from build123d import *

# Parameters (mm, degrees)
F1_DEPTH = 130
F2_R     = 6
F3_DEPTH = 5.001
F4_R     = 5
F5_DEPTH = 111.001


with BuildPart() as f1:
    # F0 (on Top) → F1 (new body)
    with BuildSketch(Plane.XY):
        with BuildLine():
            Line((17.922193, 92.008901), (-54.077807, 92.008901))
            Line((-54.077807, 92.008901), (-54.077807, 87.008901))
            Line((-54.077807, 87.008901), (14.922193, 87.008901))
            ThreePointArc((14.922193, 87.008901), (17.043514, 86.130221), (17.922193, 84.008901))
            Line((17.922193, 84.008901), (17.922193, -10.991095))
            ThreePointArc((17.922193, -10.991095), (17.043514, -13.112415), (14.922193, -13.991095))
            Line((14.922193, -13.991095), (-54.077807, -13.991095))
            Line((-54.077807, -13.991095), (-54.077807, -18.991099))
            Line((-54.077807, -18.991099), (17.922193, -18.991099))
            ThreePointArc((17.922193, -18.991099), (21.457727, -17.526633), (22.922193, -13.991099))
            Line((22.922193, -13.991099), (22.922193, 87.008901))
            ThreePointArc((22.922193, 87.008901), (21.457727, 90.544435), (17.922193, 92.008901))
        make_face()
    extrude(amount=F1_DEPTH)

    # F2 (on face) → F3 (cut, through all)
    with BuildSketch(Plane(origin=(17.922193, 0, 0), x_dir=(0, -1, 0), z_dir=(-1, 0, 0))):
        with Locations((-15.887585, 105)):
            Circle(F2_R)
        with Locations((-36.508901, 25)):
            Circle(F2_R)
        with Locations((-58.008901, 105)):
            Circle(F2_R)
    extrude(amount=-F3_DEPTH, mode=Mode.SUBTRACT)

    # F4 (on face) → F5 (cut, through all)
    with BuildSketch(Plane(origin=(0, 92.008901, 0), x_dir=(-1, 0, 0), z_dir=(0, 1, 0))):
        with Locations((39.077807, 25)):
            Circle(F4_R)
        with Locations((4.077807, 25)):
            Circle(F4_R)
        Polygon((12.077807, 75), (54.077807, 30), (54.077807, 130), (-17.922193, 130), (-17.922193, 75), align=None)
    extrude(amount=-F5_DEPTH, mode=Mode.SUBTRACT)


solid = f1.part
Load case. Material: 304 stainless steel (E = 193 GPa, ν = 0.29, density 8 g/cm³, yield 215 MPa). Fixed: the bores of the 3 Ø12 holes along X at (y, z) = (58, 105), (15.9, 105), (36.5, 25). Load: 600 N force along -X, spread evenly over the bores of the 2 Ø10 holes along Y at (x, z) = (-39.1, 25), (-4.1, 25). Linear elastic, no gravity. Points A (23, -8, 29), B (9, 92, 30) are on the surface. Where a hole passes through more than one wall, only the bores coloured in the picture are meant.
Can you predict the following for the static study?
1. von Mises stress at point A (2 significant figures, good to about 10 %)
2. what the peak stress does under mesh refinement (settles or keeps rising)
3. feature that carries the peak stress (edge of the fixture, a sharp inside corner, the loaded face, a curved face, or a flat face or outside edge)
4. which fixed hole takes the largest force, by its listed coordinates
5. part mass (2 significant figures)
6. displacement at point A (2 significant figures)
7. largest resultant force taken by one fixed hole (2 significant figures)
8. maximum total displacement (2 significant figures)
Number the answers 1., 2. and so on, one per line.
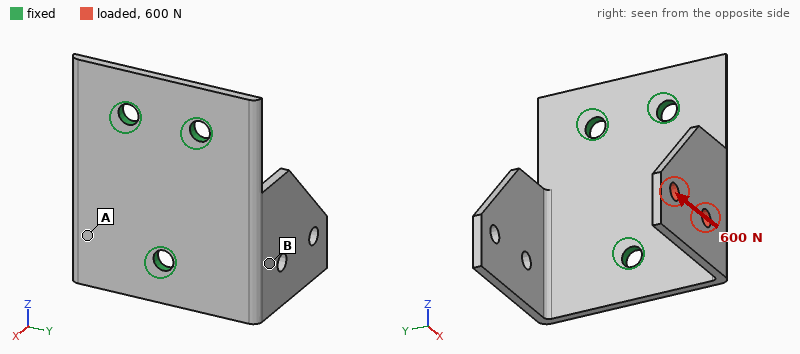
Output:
1. 23 MPa
2. keeps rising
3. edge of the fixture
4. (36.5, 25)
5. 900 g
6. 0.10 mm
7. 520 N
8. 0.35 mm
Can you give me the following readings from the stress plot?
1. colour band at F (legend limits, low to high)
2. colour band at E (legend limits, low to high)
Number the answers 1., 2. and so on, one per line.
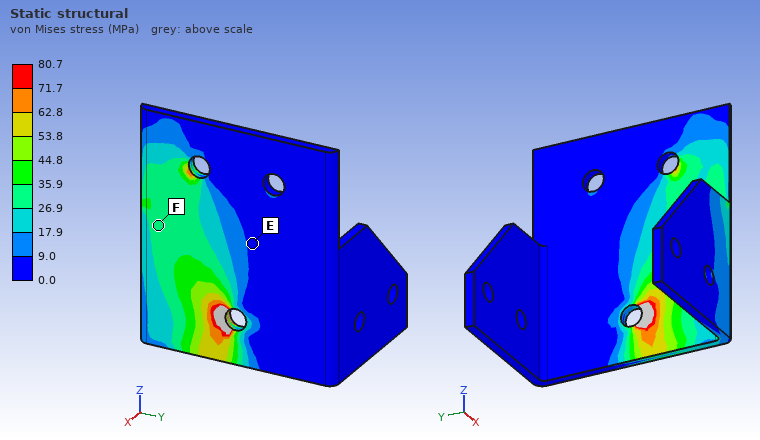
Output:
1. 26.9 to 35.9 MPa
2. 0.0 to 9.0 MPa
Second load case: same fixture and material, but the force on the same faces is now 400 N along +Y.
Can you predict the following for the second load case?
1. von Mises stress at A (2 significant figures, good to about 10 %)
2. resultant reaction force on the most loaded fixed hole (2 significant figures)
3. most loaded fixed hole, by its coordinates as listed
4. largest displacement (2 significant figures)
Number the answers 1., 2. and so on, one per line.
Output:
1. 44 MPa
2. 370 N
3. (36.5, 25)
4. 0.47 mm
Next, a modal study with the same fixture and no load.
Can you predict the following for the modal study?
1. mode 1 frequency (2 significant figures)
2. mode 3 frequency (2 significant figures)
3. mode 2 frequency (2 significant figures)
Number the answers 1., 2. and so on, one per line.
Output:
1. 470 Hz
2. 980 Hz
3. 480 Hz
